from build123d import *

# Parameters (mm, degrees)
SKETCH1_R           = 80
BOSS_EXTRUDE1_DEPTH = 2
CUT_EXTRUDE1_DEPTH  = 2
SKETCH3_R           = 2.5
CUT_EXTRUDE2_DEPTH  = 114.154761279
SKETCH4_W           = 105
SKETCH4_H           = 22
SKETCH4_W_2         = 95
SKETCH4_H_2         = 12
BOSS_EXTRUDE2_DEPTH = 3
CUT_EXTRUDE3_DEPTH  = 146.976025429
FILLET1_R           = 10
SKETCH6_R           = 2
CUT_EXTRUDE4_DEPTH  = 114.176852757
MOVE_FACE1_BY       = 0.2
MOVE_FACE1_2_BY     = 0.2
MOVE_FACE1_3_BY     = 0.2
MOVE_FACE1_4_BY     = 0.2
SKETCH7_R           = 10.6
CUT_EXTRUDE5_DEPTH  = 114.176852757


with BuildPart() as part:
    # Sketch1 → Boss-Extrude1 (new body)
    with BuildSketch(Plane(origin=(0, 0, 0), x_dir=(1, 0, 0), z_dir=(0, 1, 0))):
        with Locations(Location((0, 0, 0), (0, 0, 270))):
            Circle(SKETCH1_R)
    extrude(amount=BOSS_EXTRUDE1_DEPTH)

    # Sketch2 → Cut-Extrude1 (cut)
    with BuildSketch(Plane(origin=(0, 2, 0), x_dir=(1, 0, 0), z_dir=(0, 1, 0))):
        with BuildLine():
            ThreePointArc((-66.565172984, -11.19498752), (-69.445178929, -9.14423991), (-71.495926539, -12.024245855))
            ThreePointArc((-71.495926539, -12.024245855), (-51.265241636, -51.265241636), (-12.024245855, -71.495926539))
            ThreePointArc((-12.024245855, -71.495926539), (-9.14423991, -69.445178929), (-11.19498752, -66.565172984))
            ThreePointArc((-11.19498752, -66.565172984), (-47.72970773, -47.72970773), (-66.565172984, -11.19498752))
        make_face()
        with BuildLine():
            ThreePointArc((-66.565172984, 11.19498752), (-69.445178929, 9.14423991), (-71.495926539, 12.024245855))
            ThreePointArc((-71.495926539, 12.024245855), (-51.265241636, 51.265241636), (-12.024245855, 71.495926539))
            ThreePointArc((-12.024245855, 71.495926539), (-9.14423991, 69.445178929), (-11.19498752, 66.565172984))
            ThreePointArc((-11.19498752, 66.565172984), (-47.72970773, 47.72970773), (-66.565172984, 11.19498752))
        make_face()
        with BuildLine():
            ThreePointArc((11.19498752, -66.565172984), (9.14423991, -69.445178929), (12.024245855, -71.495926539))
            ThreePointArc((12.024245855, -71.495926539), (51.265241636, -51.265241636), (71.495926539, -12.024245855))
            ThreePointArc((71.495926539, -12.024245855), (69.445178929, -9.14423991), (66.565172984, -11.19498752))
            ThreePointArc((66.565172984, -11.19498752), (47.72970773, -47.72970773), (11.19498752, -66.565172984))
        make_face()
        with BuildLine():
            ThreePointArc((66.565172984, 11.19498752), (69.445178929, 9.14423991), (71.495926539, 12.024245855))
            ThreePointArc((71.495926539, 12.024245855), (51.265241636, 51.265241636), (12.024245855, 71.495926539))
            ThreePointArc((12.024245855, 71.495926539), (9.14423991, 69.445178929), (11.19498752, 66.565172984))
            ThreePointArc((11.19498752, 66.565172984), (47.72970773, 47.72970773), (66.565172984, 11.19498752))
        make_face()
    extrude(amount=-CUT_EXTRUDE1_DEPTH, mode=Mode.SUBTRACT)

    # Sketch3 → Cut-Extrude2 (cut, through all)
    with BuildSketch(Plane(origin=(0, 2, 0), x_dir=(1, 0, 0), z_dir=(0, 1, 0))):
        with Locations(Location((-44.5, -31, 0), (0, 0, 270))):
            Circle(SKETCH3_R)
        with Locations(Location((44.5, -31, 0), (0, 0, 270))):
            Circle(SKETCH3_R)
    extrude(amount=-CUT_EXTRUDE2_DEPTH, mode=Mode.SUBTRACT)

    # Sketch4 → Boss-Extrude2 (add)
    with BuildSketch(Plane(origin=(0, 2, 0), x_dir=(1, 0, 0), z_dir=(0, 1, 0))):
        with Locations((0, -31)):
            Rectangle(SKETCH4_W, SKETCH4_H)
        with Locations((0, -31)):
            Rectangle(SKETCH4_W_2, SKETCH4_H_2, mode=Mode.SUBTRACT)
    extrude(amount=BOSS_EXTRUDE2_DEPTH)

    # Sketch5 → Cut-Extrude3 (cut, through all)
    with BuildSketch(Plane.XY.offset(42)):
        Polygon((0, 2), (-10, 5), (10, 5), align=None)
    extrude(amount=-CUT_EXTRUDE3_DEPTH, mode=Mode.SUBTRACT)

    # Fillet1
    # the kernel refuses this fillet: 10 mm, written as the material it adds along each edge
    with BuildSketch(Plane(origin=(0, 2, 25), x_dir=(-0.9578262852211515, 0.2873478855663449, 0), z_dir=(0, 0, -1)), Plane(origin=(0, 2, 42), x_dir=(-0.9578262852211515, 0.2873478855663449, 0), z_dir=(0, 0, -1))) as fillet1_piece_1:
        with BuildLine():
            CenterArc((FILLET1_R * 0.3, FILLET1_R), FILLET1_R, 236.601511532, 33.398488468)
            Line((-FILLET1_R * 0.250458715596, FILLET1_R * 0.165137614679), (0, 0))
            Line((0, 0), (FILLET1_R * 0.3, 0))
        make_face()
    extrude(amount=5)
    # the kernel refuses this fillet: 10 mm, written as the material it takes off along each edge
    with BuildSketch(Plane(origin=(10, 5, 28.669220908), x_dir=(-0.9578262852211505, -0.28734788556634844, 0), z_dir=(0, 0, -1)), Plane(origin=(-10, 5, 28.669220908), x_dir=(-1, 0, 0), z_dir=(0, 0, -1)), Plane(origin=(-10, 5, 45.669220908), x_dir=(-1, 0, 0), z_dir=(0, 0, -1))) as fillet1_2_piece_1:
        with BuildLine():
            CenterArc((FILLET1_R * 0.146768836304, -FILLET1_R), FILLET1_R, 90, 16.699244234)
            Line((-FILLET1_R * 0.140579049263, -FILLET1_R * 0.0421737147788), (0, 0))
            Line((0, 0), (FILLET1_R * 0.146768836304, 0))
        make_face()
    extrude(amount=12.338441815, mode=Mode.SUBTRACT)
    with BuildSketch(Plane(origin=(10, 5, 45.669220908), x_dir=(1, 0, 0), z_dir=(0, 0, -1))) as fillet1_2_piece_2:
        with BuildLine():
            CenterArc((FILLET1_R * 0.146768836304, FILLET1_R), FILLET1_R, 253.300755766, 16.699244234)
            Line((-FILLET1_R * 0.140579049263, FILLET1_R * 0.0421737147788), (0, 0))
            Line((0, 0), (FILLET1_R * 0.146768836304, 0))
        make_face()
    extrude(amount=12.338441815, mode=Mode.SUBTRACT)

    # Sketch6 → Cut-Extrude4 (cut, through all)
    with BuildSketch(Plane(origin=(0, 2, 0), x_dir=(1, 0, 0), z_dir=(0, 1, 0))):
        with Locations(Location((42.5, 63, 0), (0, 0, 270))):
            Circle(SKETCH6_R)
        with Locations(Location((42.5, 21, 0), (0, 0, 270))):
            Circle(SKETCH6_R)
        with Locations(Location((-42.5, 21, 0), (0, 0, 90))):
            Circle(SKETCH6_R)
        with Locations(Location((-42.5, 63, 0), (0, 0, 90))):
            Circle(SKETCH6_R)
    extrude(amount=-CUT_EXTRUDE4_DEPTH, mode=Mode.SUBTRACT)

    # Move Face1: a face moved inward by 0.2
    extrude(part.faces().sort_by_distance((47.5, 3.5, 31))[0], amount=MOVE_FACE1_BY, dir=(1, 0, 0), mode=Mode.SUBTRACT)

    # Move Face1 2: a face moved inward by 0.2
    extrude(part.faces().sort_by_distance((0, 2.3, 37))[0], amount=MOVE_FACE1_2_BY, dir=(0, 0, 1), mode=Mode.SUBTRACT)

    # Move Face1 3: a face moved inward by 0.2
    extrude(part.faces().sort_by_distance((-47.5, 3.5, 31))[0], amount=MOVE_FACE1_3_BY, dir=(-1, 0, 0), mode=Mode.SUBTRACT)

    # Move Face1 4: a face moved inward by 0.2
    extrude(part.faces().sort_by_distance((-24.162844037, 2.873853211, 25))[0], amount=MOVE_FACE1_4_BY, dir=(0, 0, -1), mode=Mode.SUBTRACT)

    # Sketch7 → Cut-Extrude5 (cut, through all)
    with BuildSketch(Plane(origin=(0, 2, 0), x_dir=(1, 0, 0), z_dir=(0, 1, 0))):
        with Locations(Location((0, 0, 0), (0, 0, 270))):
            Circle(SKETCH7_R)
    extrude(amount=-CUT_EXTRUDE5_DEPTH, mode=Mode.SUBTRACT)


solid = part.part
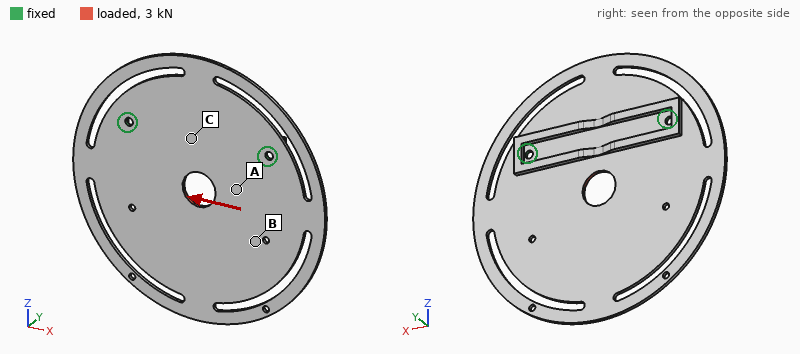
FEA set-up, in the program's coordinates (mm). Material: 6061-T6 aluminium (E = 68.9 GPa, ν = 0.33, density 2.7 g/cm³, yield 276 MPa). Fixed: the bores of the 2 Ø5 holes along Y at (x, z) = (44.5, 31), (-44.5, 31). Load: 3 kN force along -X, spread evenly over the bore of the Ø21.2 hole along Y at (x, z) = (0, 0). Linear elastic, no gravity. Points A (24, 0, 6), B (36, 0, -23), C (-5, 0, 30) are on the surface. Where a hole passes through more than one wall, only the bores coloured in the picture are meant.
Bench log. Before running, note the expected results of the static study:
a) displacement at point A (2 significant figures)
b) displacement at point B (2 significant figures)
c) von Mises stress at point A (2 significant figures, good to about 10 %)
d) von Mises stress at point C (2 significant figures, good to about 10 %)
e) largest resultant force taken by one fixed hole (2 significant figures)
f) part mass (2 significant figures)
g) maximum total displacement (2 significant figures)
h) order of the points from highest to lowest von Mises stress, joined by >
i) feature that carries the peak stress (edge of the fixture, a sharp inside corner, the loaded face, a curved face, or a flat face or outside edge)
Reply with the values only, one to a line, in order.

20 µm
31 µm
26 MPa
15 MPa
1.8 kN
100 g
38 µm
A > C > B
edge of the fixture
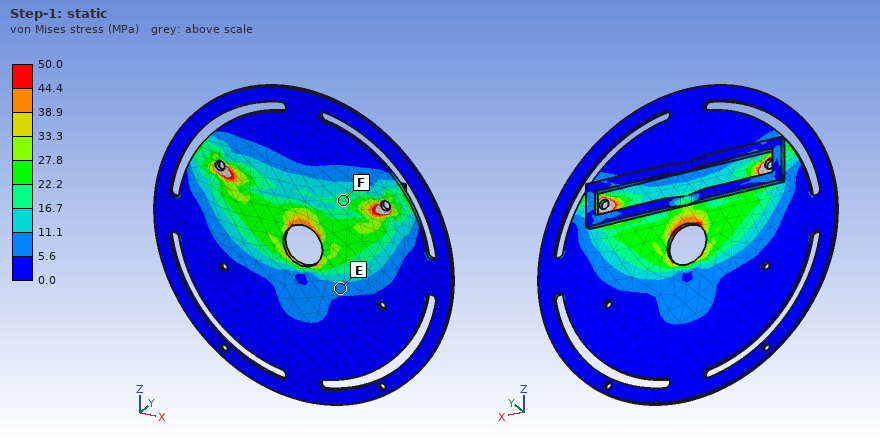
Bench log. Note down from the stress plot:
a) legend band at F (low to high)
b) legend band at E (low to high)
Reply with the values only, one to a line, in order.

16.7 to 22.2 MPa
5.6 to 11.1 MPa
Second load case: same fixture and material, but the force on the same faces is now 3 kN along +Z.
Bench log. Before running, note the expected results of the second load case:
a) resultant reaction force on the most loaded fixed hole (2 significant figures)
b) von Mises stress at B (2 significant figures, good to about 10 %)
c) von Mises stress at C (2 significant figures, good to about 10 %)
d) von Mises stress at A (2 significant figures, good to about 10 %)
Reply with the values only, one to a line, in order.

1.5 kN
8.9 MPa
12 MPa
15 MPa
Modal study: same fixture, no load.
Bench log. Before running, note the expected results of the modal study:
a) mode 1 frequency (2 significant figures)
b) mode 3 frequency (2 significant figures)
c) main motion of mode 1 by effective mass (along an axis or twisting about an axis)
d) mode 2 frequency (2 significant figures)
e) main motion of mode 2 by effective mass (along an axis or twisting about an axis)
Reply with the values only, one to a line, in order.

180 Hz
610 Hz
along Y
390 Hz
twisting about Z
